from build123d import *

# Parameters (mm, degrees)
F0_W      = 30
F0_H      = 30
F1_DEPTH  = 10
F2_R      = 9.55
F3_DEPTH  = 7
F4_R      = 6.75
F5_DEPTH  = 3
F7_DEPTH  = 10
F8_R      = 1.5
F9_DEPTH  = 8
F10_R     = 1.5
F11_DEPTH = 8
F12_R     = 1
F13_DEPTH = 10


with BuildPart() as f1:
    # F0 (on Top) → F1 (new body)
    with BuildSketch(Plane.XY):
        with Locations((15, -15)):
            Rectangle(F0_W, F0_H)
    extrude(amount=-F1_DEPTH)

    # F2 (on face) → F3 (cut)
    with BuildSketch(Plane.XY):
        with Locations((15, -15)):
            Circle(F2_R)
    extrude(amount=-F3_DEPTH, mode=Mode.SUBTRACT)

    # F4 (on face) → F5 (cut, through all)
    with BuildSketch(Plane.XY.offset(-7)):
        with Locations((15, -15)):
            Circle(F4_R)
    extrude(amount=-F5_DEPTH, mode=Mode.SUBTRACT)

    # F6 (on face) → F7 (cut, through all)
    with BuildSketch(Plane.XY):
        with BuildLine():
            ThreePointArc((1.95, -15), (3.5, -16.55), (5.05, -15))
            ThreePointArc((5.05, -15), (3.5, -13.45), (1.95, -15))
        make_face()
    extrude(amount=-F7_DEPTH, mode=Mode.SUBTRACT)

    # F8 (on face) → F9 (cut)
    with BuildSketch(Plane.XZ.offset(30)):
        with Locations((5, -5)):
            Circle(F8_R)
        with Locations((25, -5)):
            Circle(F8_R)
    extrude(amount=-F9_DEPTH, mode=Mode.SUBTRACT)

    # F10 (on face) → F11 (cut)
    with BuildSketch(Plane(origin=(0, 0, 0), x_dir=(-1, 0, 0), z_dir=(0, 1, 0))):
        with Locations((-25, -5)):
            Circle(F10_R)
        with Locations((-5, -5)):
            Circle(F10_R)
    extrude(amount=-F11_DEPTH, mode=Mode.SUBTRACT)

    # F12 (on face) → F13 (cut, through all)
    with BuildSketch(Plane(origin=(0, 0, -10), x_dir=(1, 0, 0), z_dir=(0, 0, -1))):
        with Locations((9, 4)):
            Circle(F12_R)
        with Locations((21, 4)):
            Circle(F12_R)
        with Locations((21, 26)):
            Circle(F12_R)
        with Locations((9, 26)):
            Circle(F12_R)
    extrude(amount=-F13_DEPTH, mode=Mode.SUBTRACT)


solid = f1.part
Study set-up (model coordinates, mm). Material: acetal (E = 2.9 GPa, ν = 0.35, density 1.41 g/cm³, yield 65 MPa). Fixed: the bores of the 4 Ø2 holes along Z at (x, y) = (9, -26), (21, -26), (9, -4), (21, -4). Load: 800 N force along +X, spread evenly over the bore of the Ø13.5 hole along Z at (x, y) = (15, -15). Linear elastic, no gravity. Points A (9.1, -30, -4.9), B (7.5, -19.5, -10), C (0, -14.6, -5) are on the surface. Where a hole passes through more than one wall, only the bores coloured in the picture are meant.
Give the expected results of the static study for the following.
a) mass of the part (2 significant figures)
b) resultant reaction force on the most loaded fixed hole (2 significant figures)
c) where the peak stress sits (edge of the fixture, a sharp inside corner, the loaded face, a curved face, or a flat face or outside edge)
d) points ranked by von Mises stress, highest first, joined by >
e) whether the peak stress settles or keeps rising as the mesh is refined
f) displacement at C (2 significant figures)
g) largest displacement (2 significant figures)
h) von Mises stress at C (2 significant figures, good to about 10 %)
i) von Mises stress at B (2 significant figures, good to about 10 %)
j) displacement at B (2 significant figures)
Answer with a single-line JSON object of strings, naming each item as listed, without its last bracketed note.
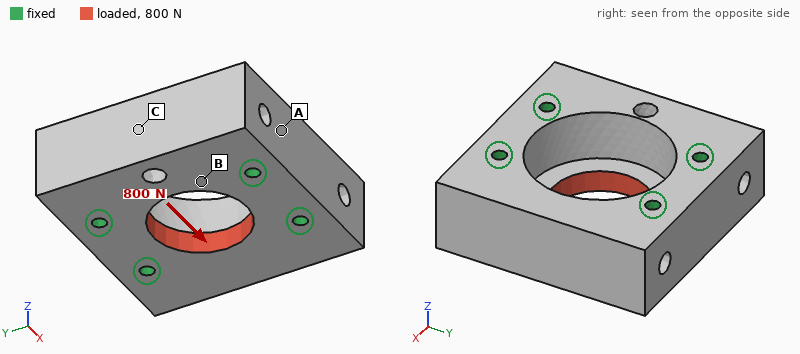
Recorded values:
{"mass of the part": "8.7 g", "resultant reaction force on the most loaded fixed hole": "200 N", "where the peak stress sits": "edge of the fixture", "points ranked by von Mises stress, highest first, joined by >": "B > C > A", "whether the peak stress settles or keeps rising as the mesh is refined": "keeps rising", "displacement at C": "19 µm", "largest displacement": "50 µm", "von Mises stress at C": "3.5 MPa", "von Mises stress at B": "6.8 MPa", "displacement at B": "31 µm"}
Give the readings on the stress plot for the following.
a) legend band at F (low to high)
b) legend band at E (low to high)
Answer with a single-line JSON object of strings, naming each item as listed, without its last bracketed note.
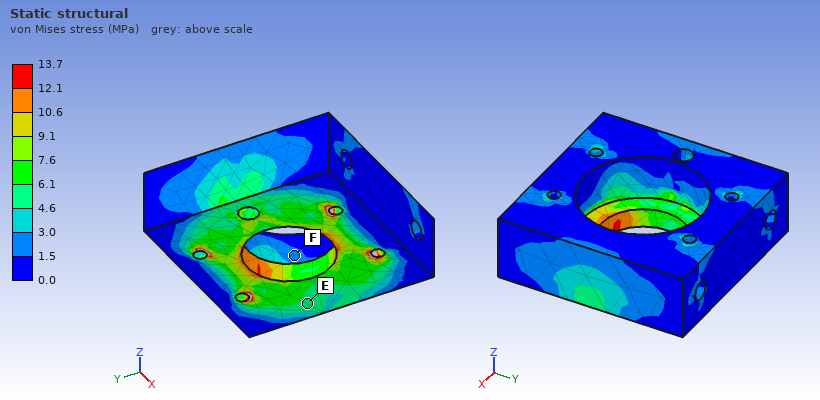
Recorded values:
{"legend band at F": "1.5 to 3.0 MPa", "legend band at E": "4.6 to 6.1 MPa"}
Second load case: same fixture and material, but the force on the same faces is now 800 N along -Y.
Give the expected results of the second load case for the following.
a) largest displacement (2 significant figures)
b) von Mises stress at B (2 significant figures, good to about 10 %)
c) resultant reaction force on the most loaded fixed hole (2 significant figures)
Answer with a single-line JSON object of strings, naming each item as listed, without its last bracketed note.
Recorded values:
{"largest displacement": "23 µm", "von Mises stress at B": "5.1 MPa", "resultant reaction force on the most loaded fixed hole": "200 N"}
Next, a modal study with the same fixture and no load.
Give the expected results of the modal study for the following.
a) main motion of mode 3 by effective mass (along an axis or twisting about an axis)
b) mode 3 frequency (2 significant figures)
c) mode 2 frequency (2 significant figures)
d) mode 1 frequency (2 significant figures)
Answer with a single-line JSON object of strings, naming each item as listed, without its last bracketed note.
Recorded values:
{"main motion of mode 3 by effective mass": "along Y", "mode 3 frequency": "14 kHz", "mode 2 frequency": "11 kHz", "mode 1 frequency": "10 kHz"}
